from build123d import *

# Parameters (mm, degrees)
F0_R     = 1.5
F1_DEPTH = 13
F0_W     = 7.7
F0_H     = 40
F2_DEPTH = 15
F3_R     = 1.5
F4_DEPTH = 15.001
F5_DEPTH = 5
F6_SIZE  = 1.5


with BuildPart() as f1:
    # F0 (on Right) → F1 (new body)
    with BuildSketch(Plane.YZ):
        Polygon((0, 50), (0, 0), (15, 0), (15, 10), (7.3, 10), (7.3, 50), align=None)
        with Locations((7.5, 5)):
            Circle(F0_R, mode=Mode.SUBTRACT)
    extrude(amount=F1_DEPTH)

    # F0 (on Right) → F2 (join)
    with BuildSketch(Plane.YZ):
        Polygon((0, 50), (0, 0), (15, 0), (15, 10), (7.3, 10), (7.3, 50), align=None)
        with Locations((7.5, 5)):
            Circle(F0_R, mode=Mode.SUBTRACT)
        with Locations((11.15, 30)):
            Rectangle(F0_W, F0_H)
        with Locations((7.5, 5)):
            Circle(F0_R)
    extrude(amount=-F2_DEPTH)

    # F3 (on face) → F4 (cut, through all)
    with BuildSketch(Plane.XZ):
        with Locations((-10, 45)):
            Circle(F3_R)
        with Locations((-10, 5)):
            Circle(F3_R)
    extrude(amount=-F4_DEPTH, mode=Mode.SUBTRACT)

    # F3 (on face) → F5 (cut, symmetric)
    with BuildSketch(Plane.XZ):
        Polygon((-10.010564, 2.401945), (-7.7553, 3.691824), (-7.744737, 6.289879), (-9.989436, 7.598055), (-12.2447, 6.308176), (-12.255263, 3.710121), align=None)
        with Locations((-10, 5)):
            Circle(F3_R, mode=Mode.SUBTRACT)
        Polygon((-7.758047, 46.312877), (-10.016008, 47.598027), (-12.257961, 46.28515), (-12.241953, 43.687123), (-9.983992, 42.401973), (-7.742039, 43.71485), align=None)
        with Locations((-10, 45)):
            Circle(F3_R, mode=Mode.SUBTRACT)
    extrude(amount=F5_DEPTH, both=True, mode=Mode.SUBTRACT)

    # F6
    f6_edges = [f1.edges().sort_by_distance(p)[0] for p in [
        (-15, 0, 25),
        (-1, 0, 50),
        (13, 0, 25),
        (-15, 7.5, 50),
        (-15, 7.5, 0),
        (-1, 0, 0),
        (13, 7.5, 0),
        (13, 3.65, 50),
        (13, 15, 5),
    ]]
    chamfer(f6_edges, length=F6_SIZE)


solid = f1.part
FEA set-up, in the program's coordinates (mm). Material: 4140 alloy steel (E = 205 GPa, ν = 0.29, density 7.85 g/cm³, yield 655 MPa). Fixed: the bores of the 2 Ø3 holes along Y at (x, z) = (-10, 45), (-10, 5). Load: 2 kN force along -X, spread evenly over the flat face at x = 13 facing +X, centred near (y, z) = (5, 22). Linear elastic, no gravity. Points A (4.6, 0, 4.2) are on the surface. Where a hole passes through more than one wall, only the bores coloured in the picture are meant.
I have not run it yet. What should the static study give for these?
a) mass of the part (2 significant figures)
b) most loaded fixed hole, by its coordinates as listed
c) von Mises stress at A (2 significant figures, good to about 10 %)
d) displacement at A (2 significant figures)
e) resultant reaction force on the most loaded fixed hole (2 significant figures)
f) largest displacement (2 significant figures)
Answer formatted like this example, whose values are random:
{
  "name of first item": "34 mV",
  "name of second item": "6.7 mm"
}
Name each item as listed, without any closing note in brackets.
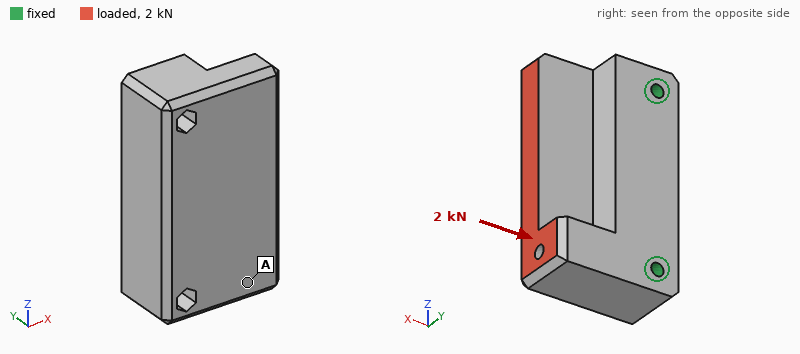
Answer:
{
  "mass of the part": "130 g",
  "most loaded fixed hole, by its coordinates as listed": "(-10, 5)",
  "von Mises stress at A": "4.9 MPa",
  "displacement at A": "1.9 µm",
  "resultant reaction force on the most loaded fixed hole": "1.2 kN",
  "largest displacement": "2.9 µm"
}
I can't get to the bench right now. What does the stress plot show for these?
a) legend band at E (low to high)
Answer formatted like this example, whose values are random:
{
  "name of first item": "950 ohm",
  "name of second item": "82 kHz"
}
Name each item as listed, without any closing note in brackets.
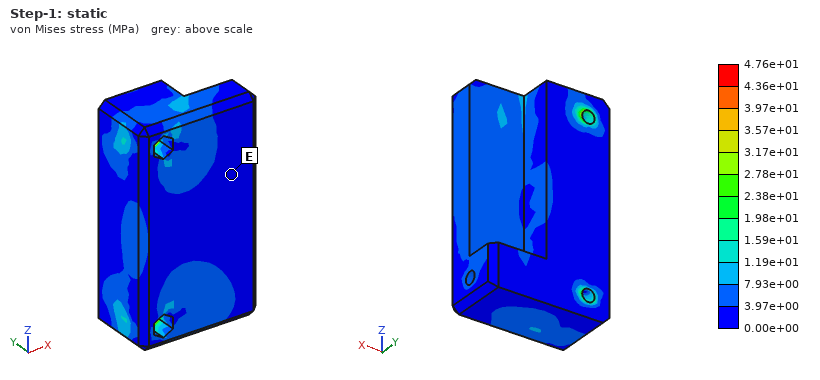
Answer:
{
  "legend band at E": "0.00e+00 to 3.97e+00 MPa"
}
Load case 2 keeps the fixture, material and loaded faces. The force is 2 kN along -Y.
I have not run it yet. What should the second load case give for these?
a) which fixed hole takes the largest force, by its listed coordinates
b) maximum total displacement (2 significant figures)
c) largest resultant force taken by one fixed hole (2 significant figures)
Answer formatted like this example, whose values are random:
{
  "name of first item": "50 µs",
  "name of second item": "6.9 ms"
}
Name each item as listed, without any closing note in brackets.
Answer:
{
  "which fixed hole takes the largest force, by its listed coordinates": "(-10, 5)",
  "maximum total displacement": "22 µm",
  "largest resultant force taken by one fixed hole": "1.1 kN"
}
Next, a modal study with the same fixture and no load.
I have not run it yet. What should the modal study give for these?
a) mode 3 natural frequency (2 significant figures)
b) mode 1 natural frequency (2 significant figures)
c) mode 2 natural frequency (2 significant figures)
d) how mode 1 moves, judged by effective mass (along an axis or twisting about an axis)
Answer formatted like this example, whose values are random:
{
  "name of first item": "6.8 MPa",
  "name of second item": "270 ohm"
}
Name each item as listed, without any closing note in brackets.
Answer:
{
  "mode 3 natural frequency": "22 kHz",
  "mode 1 natural frequency": "10 kHz",
  "mode 2 natural frequency": "17 kHz",
  "how mode 1 moves, judged by effective mass": "along Y"
}
